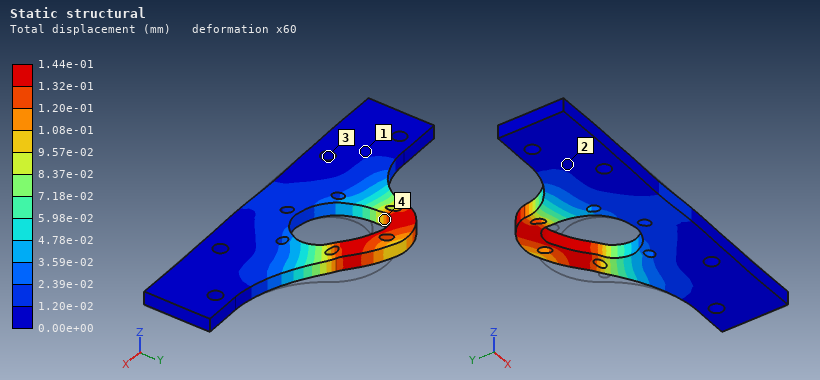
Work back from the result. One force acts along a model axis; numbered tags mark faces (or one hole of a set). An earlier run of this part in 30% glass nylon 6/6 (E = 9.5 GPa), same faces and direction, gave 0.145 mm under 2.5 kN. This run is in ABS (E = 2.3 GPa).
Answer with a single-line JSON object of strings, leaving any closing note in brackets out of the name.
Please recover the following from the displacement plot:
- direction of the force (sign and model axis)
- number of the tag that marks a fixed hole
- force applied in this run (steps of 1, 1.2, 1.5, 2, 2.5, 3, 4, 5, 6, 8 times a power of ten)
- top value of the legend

{"direction of the force": "-X", "number of the tag that marks a fixed hole": "3", "force applied in this run": "600 N", "top value of the legend": "1.44e-01 mm"}
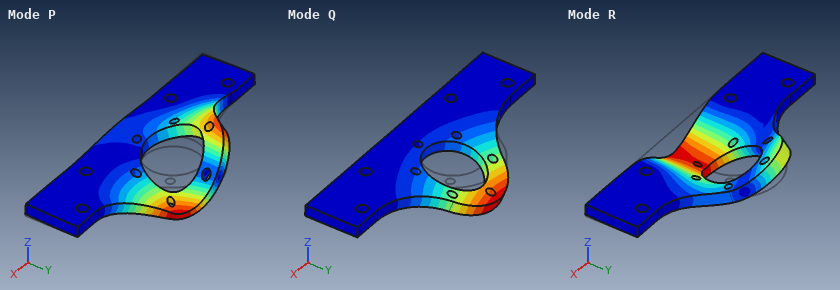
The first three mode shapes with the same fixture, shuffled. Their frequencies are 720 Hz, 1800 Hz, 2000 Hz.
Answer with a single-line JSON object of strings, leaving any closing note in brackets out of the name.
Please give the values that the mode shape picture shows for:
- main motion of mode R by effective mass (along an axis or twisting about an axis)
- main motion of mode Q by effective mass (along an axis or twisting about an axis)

{"main motion of mode R by effective mass": "along Z", "main motion of mode Q by effective mass": "along Z"}
